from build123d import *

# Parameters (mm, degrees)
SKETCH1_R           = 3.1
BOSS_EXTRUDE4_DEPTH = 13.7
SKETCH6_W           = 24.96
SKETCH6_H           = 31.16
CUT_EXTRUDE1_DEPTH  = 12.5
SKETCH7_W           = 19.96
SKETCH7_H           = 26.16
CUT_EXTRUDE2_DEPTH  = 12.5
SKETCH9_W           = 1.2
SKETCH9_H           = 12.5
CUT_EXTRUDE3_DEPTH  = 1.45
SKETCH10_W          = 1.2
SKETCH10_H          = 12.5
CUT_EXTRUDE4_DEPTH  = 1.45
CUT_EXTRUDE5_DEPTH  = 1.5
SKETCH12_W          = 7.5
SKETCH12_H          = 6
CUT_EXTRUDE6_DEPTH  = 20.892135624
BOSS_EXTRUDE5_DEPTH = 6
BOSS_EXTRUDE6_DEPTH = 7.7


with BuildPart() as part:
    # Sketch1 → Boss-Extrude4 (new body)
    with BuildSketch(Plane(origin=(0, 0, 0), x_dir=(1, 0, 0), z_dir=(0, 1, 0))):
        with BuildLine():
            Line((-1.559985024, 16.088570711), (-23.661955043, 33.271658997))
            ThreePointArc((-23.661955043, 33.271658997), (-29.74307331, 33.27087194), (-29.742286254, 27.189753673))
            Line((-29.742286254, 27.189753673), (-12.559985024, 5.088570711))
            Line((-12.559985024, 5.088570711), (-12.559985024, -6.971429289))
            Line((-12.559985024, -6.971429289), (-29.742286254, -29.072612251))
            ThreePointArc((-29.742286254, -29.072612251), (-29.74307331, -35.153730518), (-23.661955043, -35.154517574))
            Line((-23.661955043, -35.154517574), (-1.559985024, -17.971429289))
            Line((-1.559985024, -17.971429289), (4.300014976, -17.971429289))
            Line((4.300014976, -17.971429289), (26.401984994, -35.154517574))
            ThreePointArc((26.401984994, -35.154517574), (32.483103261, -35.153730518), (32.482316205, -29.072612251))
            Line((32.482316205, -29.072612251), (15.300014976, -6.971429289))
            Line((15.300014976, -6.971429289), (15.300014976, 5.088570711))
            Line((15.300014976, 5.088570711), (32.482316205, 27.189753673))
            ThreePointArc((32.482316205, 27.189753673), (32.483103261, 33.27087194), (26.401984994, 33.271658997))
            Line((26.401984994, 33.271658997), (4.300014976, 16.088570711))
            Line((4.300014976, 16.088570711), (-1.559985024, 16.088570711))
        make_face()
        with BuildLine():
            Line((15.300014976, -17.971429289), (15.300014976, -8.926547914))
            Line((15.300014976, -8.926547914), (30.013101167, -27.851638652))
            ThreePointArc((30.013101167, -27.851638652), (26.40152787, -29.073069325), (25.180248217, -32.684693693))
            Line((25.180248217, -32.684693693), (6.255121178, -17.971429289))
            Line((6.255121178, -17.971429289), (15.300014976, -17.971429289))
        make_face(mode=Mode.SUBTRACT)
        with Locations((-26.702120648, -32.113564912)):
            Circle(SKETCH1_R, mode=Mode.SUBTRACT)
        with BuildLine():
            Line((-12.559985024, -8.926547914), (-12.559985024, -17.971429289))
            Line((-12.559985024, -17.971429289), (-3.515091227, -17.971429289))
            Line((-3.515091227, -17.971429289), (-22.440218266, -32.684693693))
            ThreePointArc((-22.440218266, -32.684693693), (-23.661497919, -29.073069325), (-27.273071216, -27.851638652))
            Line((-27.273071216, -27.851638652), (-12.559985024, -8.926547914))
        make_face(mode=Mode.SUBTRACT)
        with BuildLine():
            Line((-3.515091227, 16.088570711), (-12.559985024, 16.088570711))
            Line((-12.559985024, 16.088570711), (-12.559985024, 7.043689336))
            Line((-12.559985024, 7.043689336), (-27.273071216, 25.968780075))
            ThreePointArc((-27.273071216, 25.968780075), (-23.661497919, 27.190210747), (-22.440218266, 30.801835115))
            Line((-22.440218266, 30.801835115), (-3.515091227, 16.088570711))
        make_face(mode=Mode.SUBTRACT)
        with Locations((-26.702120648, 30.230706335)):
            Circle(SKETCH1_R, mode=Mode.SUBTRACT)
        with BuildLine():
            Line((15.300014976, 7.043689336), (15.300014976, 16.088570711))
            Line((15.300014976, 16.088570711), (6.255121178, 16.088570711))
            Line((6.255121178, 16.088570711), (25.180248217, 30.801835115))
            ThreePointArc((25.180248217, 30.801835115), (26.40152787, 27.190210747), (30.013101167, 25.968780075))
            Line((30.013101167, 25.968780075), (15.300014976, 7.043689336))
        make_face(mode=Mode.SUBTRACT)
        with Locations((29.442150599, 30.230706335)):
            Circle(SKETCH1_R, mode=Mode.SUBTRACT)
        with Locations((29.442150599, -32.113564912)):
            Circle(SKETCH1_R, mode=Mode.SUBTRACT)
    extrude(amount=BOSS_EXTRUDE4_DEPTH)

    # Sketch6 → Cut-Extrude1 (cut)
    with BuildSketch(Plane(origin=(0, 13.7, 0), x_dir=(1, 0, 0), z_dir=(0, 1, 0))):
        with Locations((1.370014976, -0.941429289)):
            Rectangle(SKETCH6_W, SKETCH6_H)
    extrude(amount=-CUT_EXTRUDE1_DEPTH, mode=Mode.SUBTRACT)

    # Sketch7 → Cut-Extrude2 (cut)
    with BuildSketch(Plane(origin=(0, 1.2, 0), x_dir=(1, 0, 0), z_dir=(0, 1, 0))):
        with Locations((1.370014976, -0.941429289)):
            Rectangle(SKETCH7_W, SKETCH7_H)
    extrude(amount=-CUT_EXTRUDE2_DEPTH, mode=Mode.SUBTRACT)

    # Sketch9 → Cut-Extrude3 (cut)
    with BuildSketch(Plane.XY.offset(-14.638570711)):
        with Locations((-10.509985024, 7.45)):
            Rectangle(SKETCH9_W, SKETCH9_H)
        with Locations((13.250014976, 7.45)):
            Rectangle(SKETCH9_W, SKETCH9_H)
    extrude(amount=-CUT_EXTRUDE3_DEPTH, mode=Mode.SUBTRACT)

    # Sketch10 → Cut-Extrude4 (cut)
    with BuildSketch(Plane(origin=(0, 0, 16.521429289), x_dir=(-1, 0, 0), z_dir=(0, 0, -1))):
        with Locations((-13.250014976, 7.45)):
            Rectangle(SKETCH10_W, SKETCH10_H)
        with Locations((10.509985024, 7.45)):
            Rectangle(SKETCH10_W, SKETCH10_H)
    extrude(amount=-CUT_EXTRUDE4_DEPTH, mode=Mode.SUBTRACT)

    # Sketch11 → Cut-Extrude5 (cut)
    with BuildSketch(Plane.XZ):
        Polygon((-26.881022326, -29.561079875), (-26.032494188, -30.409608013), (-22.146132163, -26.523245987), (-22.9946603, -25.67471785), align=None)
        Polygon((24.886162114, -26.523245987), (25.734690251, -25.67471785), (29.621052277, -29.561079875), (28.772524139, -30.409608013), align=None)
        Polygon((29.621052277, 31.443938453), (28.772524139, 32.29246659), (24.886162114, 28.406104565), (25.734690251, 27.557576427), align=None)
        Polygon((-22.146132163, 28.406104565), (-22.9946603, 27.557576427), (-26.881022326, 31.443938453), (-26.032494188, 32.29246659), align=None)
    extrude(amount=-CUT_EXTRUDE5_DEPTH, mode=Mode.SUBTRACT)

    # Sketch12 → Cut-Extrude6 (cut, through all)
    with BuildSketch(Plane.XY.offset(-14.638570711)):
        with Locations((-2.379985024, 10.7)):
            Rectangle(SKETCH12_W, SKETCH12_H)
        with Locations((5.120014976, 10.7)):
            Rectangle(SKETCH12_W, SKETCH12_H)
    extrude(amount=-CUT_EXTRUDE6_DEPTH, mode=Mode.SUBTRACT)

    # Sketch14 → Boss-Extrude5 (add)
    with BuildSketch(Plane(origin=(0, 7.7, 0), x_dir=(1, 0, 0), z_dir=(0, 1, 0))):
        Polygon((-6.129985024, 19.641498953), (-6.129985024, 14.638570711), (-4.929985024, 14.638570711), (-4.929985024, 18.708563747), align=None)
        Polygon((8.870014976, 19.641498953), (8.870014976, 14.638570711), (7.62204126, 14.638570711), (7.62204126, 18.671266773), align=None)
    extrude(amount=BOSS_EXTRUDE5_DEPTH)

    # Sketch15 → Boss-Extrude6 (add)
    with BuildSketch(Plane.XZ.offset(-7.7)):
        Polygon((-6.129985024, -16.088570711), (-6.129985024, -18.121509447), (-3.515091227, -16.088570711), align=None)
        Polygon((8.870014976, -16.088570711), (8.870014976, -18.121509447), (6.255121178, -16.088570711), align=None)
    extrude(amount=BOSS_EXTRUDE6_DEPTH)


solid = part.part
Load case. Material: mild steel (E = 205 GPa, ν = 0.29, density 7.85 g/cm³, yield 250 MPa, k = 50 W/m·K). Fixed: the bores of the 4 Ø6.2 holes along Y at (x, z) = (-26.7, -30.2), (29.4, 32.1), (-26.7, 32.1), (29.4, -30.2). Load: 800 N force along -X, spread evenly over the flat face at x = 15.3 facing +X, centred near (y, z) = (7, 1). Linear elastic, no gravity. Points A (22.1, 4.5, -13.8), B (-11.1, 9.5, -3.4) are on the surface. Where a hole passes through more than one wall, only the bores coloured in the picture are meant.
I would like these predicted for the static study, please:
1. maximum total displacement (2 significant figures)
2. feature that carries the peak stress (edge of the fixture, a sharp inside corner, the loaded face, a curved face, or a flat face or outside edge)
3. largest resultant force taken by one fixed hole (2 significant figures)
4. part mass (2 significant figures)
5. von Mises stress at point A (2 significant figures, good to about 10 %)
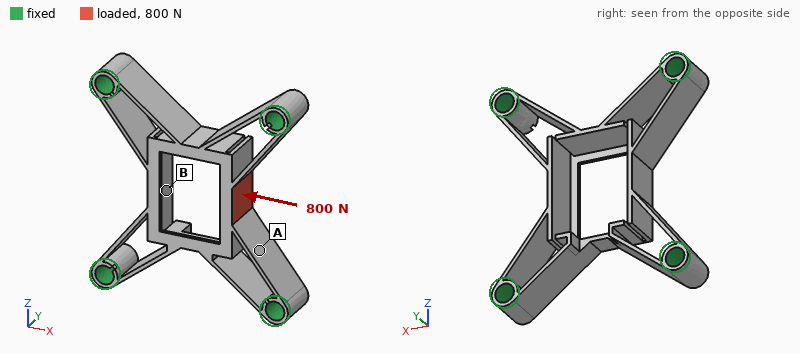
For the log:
26 µm
a flat face or outside edge
630 N
58 g
49 MPa
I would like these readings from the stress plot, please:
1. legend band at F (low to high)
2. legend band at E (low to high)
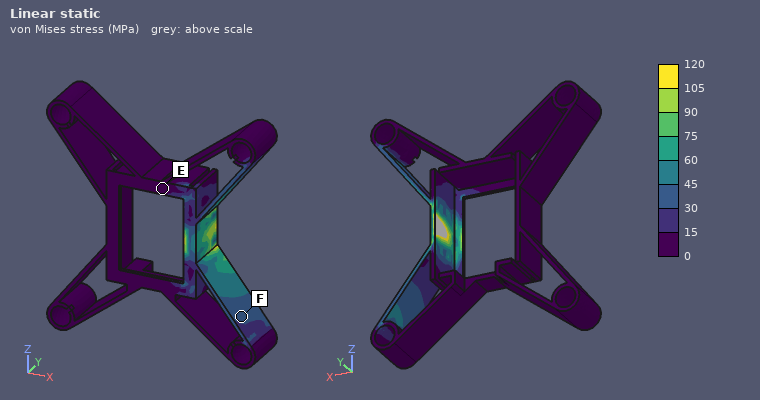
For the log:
30 to 45 MPa
0 to 15 MPa
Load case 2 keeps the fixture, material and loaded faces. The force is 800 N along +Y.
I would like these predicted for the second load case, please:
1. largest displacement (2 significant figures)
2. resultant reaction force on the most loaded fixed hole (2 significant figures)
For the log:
37 µm
400 N
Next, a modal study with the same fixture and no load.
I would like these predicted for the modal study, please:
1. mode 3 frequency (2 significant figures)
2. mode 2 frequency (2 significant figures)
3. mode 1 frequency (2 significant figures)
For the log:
6900 Hz
6200 Hz
6000 Hz
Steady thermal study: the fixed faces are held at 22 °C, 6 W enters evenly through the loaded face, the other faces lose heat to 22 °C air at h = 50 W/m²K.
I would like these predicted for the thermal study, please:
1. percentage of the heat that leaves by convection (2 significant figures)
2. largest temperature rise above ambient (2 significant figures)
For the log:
60 %
44 K
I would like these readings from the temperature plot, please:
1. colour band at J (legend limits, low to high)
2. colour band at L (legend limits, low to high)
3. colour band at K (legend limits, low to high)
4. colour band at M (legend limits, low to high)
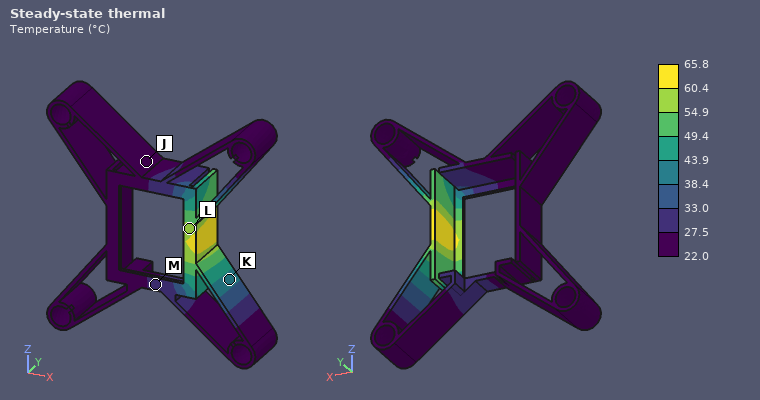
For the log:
22.0 to 27.5 °C
54.9 to 60.4 °C
38.4 to 43.9 °C
27.5 to 33.0 °C
